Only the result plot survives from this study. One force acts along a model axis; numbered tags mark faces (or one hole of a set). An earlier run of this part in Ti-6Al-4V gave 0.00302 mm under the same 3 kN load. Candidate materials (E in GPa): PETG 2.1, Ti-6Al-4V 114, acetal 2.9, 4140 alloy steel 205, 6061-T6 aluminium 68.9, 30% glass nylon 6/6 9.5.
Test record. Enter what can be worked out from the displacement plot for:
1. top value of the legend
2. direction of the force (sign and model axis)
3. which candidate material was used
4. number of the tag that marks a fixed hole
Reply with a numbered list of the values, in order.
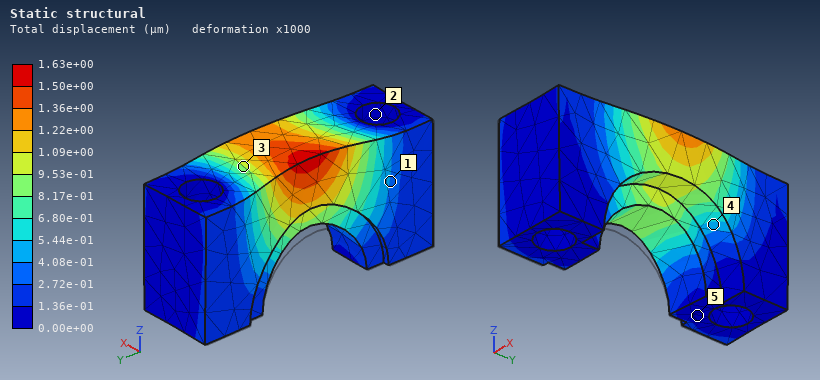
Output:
1. 1.63e+00 µm
2. +X
3. 4140 alloy steel
4. 2
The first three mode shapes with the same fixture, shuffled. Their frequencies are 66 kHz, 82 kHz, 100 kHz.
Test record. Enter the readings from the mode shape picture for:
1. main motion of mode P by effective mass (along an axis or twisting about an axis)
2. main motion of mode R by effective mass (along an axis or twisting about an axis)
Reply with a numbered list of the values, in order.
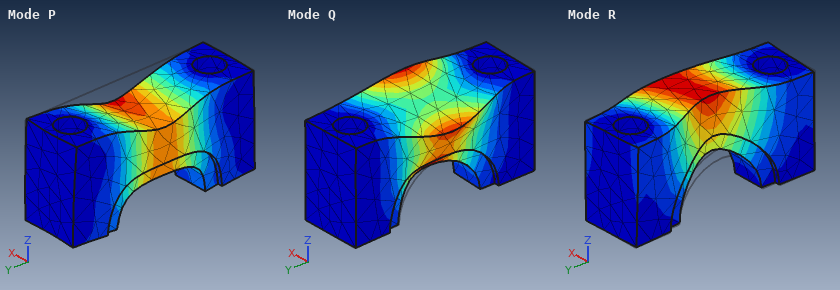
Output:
1. along Z
2. along X
